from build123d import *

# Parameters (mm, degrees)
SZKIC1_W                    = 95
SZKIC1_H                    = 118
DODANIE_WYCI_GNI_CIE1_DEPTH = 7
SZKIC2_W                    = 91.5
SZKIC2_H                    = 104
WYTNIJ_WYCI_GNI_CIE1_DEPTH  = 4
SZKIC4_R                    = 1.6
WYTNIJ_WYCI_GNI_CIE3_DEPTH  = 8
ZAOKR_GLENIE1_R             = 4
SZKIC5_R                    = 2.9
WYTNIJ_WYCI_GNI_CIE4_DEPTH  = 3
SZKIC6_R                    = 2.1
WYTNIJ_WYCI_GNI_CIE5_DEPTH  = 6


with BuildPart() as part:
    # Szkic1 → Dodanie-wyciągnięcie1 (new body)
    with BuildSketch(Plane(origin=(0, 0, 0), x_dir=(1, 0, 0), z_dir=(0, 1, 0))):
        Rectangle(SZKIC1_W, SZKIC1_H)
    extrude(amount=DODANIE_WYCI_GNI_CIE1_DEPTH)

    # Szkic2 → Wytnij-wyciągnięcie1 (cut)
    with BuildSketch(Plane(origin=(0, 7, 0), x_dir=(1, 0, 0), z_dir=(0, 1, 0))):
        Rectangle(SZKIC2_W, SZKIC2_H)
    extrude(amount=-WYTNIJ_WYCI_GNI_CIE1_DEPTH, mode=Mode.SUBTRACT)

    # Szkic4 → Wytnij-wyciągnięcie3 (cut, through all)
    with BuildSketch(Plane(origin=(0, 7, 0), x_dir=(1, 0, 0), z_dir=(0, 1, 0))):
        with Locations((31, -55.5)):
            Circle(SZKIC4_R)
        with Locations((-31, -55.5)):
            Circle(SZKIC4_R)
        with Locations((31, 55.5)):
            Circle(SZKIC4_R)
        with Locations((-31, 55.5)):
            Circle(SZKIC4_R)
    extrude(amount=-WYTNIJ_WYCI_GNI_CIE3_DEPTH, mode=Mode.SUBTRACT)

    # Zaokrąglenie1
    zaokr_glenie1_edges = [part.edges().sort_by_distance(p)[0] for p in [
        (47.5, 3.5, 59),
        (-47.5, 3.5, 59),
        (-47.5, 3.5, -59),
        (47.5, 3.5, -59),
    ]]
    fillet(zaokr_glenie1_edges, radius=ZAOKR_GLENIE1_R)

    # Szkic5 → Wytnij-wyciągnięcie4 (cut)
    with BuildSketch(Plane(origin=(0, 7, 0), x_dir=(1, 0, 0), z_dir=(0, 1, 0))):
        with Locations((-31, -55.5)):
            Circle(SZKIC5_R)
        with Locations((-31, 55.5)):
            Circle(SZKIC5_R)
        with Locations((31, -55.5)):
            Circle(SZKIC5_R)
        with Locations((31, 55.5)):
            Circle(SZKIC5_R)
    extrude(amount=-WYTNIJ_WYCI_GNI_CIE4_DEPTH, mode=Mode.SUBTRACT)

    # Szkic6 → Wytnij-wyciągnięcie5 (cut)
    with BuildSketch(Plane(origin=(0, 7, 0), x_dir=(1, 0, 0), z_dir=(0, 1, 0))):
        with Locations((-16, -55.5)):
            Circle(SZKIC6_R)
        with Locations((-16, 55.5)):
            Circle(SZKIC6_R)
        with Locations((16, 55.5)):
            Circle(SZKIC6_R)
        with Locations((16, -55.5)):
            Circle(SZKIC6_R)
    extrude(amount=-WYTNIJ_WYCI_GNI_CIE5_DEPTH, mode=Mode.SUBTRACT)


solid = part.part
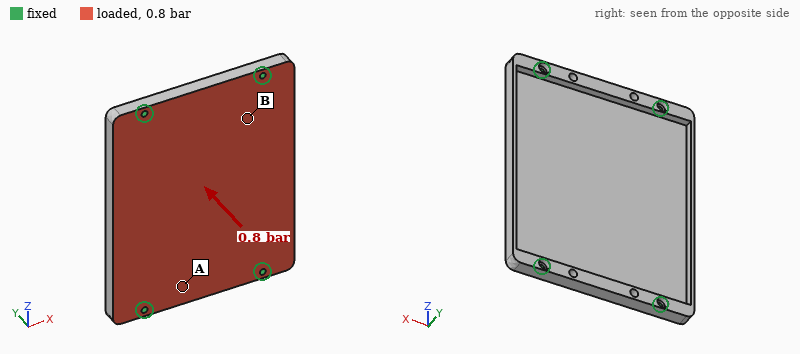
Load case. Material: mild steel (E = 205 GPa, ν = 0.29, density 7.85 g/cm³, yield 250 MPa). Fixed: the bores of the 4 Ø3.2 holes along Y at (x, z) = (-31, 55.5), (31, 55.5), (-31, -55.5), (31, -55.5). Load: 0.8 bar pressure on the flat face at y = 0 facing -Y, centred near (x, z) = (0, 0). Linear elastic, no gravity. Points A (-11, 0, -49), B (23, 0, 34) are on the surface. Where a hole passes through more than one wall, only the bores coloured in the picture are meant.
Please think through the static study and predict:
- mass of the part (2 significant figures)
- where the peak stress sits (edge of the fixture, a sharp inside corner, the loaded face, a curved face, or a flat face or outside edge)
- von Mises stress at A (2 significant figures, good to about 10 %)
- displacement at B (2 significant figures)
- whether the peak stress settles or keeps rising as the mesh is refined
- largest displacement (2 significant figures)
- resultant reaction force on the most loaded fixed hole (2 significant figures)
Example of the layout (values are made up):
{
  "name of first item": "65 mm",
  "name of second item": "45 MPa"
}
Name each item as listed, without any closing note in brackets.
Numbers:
{
  "mass of the part": "310 g",
  "where the peak stress sits": "edge of the fixture",
  "von Mises stress at A": "17 MPa",
  "displacement at B": "26 µm",
  "whether the peak stress settles or keeps rising as the mesh is refined": "keeps rising",
  "largest displacement": "63 µm",
  "resultant reaction force on the most loaded fixed hole": "240 N"
}
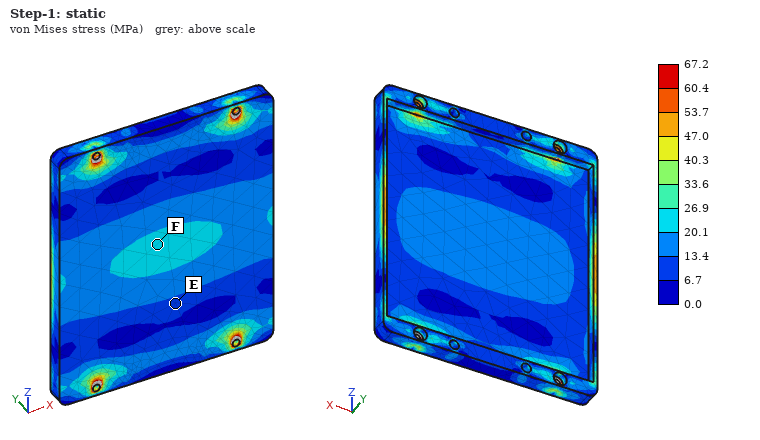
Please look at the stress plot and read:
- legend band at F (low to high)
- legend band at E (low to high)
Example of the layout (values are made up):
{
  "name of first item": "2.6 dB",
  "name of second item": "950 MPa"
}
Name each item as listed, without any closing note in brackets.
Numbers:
{
  "legend band at F": "20.1 to 26.9 MPa",
  "legend band at E": "6.7 to 13.4 MPa"
}
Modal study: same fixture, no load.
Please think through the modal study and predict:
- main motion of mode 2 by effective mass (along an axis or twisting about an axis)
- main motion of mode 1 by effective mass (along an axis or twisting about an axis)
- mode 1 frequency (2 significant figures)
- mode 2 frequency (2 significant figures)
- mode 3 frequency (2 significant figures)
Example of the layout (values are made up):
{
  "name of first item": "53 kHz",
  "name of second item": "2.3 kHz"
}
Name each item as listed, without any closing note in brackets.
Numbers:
{
  "main motion of mode 2 by effective mass": "twisting about Z",
  "main motion of mode 1 by effective mass": "along Y",
  "mode 1 frequency": "1400 Hz",
  "mode 2 frequency": "1900 Hz",
  "mode 3 frequency": "2800 Hz"
}
